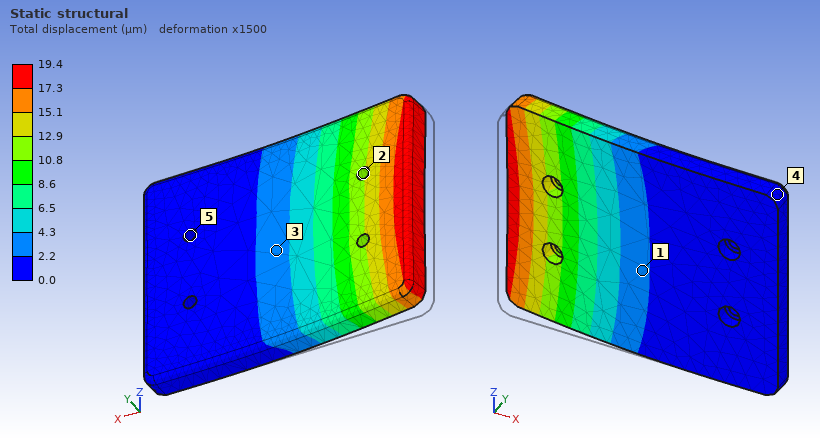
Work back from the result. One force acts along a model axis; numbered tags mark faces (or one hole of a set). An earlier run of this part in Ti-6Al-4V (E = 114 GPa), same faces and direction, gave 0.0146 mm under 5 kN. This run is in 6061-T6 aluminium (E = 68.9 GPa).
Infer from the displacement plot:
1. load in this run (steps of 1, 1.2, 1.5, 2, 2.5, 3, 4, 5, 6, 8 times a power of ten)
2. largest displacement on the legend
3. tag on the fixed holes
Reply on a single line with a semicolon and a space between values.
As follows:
4 kN; 19.4 µm; 5
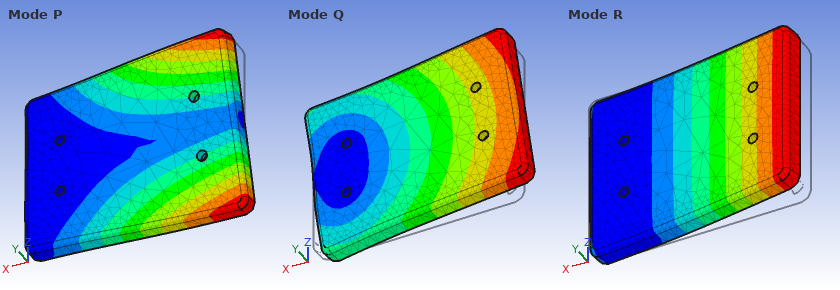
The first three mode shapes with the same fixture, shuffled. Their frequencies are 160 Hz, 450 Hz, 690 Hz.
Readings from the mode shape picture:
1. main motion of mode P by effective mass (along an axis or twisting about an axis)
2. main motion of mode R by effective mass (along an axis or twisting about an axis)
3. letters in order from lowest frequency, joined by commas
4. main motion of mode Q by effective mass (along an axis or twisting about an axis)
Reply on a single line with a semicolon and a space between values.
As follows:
twisting about X; along Y; R, P, Q; along Z
